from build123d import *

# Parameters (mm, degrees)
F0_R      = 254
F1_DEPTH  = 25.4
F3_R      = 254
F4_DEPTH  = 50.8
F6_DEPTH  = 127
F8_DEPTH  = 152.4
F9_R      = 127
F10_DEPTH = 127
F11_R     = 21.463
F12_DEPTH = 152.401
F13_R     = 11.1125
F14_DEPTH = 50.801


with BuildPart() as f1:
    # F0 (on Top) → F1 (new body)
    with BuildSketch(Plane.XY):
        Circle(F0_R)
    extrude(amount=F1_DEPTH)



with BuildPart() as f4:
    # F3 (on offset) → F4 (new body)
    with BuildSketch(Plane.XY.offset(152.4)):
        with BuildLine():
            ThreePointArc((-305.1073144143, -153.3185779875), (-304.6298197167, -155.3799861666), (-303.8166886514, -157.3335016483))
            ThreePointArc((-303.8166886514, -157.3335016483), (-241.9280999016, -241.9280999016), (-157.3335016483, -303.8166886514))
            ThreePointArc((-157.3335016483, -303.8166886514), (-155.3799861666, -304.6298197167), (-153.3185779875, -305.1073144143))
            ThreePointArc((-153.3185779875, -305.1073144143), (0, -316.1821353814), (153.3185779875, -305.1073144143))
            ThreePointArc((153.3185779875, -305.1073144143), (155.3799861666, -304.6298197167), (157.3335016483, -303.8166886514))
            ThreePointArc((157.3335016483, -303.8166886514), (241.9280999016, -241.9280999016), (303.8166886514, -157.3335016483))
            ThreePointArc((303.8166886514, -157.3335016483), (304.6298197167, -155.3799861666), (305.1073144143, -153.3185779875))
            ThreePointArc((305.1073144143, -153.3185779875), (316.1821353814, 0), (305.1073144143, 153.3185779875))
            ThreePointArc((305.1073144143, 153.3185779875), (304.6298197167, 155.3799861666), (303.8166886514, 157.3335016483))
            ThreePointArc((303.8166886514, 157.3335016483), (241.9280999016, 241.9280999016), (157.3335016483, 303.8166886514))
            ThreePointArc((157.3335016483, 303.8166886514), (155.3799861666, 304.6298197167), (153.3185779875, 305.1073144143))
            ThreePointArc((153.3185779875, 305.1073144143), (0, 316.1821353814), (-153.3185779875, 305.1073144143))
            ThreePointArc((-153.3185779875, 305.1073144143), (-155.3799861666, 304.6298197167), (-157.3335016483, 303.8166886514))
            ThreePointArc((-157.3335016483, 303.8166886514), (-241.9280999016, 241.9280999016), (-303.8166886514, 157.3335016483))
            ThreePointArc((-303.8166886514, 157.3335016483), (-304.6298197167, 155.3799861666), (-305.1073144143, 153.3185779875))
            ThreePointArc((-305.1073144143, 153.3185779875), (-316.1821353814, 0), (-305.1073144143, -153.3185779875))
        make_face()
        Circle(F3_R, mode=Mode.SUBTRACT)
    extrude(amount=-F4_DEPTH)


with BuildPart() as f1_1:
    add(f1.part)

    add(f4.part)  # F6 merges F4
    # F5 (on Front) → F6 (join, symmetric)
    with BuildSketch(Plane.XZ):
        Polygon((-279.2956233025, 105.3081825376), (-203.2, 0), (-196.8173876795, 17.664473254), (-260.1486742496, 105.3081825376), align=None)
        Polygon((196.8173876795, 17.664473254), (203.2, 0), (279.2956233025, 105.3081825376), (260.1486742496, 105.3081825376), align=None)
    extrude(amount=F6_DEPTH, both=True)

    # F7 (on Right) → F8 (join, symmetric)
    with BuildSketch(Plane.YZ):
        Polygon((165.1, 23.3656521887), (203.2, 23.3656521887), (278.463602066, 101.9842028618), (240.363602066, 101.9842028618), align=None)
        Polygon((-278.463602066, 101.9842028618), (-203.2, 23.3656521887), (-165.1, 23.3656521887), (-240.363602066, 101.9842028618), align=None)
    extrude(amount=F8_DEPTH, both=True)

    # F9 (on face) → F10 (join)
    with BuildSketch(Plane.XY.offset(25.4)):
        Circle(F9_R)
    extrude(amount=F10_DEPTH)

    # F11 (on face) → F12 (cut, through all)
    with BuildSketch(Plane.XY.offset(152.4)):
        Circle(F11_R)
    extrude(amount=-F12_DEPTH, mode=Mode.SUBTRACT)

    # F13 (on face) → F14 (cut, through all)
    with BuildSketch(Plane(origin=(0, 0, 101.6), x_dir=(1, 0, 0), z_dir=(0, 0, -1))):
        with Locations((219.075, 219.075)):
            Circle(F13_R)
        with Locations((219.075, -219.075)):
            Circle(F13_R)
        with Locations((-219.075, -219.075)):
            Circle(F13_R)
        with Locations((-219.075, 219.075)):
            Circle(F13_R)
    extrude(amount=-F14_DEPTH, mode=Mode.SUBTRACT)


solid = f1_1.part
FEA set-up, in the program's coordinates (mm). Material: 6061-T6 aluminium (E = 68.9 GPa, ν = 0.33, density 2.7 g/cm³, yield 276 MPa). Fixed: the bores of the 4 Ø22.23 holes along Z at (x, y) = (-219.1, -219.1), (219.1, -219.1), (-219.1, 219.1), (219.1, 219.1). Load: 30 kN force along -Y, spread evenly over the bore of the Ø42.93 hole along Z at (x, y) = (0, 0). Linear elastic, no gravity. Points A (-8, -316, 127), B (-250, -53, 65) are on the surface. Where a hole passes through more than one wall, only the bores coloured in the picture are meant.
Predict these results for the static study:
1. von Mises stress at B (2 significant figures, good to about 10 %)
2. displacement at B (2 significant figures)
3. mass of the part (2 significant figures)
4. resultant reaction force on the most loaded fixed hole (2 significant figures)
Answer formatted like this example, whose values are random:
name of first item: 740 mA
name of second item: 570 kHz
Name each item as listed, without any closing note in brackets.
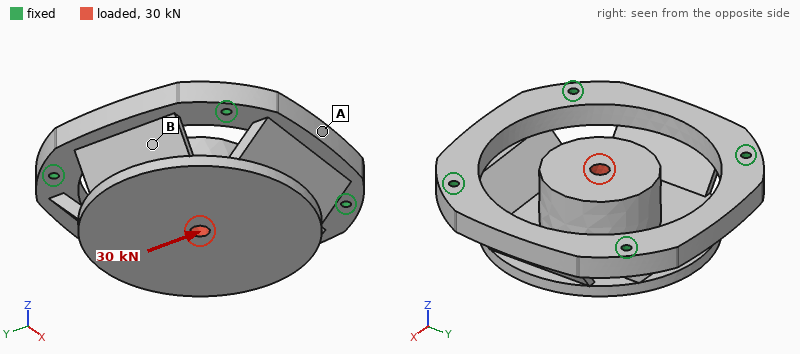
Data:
von Mises stress at B: 6.8 MPa
displacement at B: 16 µm
mass of the part: 57 kg
resultant reaction force on the most loaded fixed hole: 8.0 kN
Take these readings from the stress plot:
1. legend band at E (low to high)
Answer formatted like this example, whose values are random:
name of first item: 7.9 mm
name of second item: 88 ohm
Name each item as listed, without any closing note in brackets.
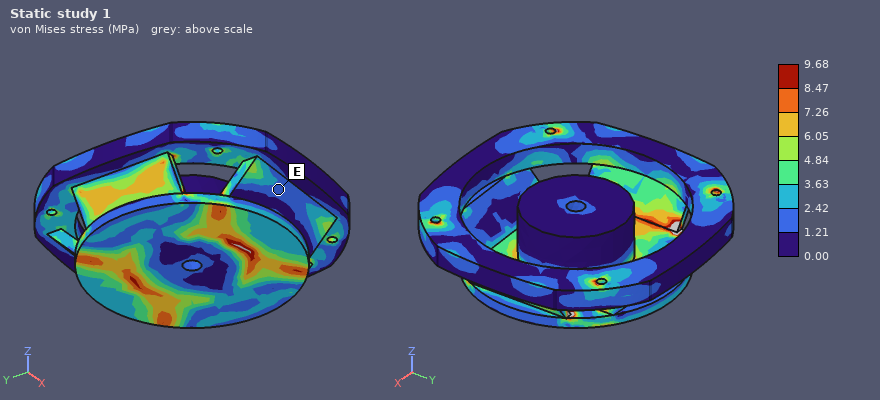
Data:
legend band at E: 1.21 to 2.42 MPa
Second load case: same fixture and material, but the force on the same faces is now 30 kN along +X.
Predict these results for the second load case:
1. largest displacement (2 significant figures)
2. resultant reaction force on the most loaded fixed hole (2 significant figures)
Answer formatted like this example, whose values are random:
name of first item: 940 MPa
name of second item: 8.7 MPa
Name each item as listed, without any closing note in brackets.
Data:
largest displacement: 72 µm
resultant reaction force on the most loaded fixed hole: 7.8 kN
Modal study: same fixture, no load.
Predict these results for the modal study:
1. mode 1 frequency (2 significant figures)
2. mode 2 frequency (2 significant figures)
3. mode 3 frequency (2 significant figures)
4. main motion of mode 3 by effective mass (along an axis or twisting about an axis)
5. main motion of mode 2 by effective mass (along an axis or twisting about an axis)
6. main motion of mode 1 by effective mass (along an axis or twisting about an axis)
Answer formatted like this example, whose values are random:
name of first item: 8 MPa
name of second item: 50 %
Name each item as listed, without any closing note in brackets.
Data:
mode 1 frequency: 620 Hz
mode 2 frequency: 650 Hz
mode 3 frequency: 750 Hz
main motion of mode 3 by effective mass: along X
main motion of mode 2 by effective mass: along Y
main motion of mode 1 by effective mass: along Z
